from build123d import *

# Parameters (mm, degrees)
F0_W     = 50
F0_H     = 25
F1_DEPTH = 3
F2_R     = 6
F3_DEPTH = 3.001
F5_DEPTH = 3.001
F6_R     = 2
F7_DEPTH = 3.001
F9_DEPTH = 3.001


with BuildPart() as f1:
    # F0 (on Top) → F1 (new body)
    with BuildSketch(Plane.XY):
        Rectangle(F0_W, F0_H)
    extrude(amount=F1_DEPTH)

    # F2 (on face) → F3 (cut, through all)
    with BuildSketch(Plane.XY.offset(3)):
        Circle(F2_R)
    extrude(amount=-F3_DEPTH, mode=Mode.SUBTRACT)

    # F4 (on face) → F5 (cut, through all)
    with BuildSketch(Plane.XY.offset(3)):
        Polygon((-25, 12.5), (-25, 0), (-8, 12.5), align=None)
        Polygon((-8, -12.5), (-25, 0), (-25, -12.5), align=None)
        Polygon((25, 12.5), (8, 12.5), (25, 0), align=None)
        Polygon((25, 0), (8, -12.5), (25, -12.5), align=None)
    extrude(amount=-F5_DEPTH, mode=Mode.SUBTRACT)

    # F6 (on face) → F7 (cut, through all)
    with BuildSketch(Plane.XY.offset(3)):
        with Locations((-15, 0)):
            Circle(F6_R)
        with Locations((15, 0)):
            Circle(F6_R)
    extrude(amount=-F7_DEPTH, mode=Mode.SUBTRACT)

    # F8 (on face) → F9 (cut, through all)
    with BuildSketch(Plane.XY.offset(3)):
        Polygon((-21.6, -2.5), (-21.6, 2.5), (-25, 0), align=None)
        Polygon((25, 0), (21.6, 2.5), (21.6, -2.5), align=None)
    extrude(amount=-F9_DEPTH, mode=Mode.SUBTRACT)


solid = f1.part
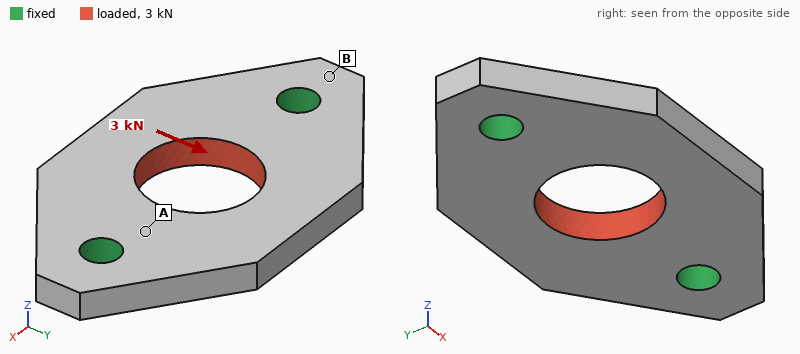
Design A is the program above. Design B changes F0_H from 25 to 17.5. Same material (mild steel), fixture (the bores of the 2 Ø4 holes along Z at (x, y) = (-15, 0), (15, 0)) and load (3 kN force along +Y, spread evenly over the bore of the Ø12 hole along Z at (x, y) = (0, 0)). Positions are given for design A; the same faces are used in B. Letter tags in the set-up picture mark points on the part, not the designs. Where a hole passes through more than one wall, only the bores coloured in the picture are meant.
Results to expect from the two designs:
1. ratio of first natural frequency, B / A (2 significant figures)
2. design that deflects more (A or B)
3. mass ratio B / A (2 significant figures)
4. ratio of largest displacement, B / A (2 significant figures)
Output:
1.6
B
0.76
1.8
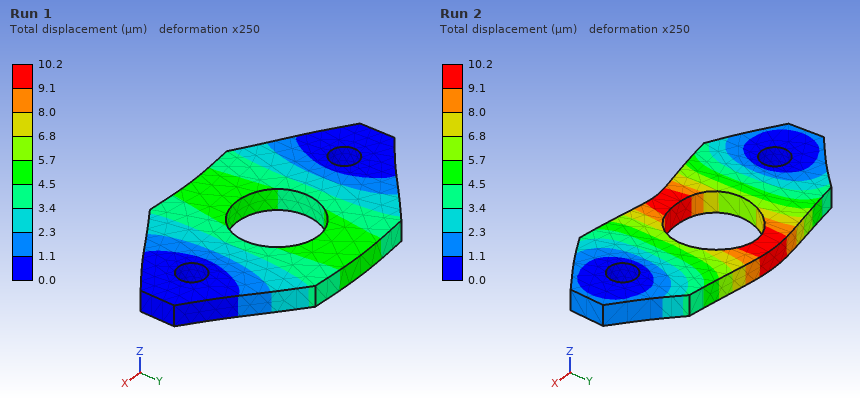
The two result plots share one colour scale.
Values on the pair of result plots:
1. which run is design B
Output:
Run 2
